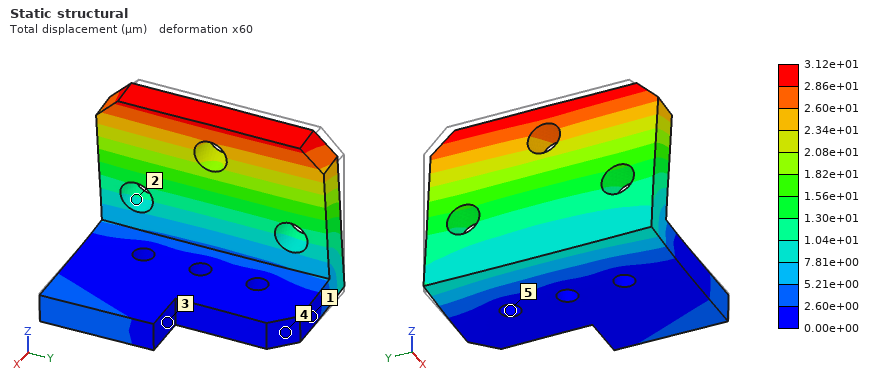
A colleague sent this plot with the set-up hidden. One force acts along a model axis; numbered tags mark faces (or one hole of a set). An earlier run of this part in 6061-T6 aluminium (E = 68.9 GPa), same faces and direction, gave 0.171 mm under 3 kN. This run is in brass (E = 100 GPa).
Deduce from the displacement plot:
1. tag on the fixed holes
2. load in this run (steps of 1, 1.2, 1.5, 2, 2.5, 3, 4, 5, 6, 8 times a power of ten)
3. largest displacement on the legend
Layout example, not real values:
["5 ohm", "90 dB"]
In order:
["5", "800 N", "3.12e+01 µm"]
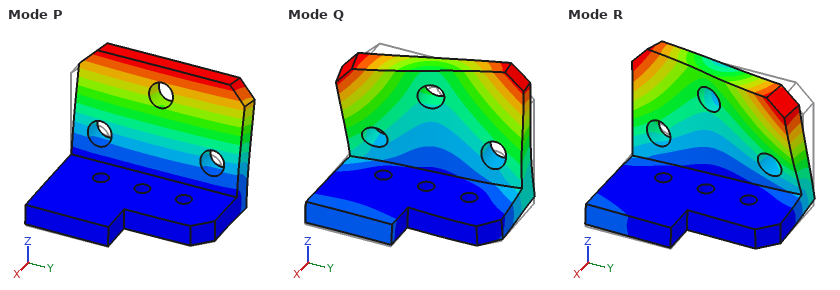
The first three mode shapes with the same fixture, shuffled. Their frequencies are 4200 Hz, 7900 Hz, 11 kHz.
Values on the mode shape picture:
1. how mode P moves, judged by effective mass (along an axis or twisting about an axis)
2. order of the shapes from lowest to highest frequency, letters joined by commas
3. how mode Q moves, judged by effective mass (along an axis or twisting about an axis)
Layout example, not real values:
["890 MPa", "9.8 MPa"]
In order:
["along X", "P, R, Q", "along Y"]
